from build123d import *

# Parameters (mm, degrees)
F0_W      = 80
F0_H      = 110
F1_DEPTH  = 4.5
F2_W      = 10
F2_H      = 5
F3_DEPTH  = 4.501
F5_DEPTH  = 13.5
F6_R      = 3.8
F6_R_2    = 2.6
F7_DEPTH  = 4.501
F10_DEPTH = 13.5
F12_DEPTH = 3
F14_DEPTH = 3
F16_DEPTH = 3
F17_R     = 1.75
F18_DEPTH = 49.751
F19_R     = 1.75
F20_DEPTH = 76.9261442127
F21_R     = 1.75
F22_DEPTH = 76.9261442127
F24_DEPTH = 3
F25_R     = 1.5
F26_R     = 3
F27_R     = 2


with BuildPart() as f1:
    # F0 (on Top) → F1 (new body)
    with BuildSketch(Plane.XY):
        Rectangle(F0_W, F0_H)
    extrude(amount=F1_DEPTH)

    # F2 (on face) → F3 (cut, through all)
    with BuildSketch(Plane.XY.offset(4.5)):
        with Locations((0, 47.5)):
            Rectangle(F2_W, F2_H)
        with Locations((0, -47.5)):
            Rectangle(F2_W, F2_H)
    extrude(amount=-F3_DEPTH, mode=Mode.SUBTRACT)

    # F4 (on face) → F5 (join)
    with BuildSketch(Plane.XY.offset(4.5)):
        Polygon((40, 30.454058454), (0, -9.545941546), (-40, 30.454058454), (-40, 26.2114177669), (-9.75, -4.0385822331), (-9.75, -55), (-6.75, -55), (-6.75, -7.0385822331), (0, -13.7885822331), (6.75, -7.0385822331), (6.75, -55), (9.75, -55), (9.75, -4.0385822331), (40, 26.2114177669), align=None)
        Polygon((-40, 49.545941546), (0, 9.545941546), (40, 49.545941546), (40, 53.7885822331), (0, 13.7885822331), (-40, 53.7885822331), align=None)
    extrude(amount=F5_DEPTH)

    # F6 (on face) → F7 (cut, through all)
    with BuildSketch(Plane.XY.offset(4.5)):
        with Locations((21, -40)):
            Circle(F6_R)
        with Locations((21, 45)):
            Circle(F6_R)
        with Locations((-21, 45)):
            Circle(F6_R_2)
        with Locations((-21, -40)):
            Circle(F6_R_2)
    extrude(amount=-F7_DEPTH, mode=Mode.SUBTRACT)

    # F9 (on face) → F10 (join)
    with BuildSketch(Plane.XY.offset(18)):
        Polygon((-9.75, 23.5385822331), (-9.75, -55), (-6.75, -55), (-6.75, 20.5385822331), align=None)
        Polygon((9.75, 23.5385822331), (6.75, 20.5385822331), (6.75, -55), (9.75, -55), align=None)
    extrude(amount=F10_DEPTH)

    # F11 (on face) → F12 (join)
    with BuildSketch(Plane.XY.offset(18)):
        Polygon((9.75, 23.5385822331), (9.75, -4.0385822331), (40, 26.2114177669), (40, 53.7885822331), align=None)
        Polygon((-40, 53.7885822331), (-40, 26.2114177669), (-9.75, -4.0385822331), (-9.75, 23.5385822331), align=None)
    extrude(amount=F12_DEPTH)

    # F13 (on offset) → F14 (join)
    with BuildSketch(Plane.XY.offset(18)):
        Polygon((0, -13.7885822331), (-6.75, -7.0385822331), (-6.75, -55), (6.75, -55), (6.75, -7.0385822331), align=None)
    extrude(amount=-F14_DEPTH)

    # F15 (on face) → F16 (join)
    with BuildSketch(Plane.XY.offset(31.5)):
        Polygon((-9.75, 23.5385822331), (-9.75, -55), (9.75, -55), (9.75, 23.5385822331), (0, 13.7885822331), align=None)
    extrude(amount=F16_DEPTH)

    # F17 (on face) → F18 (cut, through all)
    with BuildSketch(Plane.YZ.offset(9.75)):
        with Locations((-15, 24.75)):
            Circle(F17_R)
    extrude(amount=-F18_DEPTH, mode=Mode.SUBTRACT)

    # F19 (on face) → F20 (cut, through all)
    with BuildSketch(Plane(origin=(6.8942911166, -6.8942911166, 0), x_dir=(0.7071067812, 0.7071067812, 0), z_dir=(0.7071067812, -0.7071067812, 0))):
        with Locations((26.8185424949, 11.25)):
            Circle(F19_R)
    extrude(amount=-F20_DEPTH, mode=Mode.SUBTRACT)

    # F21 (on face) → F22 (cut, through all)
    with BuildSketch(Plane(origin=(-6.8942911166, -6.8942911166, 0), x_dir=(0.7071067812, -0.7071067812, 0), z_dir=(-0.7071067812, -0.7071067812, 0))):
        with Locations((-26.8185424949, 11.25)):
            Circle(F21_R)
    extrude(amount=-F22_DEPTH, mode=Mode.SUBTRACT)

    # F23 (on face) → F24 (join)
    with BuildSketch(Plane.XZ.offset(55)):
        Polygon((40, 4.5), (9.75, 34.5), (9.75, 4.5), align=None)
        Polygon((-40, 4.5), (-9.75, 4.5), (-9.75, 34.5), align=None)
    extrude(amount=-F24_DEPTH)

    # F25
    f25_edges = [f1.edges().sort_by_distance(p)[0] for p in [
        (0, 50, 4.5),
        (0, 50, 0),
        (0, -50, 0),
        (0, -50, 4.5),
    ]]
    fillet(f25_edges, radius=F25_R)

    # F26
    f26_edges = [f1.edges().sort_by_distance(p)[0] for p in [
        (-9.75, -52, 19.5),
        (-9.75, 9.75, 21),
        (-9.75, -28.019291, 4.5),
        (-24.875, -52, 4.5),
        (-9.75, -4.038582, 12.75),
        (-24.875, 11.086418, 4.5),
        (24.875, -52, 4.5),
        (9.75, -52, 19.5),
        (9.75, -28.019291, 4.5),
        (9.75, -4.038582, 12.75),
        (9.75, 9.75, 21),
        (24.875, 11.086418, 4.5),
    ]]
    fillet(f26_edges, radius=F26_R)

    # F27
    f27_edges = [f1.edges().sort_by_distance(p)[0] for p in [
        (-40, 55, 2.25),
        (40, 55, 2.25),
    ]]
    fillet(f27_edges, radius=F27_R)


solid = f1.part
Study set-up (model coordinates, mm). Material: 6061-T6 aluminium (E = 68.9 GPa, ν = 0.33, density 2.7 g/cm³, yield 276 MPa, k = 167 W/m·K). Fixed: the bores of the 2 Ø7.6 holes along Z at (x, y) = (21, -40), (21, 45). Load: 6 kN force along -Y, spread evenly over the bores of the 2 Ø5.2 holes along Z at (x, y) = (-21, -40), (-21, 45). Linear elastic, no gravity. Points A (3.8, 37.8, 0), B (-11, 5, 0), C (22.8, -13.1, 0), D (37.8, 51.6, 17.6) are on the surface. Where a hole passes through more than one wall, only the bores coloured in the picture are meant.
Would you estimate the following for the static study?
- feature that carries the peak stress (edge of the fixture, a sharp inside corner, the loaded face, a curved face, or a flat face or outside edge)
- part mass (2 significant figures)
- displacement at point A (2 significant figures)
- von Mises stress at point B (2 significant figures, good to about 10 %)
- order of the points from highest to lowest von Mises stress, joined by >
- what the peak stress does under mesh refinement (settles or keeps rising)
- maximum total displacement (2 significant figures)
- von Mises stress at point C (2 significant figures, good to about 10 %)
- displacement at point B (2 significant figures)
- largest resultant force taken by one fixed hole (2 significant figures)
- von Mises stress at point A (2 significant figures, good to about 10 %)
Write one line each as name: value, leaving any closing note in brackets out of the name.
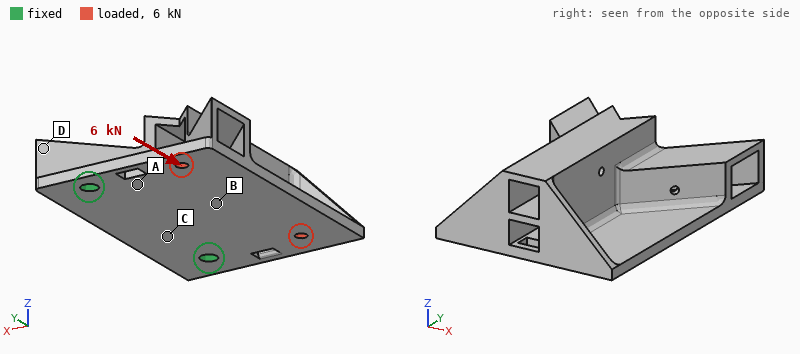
feature that carries the peak stress: edge of the fixture
part mass: 200 g
displacement at point A: 13 µm
von Mises stress at point B: 22 MPa
order of the points from highest to lowest von Mises stress, joined by >: A > B > C > D
what the peak stress does under mesh refinement: keeps rising
maximum total displacement: 54 µm
von Mises stress at point C: 12 MPa
displacement at point B: 22 µm
largest resultant force taken by one fixed hole: 4.2 kN
von Mises stress at point A: 33 MPa
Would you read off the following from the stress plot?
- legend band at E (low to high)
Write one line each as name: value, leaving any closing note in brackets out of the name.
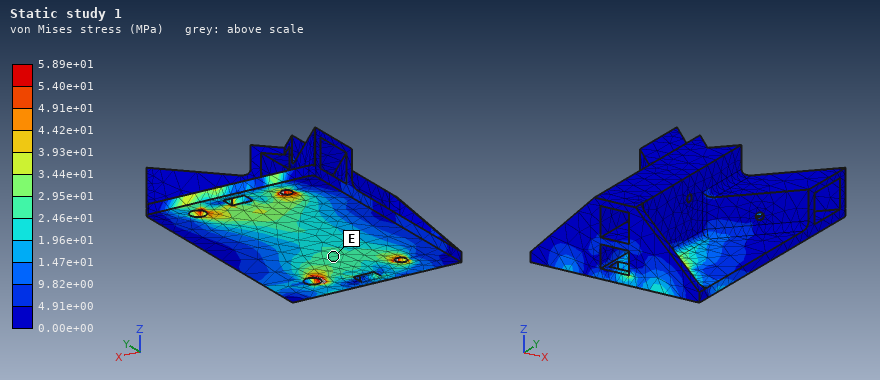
legend band at E: 2.46e+01 to 2.95e+01 MPa
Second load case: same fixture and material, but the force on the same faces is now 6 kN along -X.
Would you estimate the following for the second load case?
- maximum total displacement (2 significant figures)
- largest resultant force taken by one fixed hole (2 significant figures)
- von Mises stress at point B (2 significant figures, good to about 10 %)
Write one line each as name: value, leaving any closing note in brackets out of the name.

maximum total displacement: 26 µm
largest resultant force taken by one fixed hole: 3.0 kN
von Mises stress at point B: 4.3 MPa
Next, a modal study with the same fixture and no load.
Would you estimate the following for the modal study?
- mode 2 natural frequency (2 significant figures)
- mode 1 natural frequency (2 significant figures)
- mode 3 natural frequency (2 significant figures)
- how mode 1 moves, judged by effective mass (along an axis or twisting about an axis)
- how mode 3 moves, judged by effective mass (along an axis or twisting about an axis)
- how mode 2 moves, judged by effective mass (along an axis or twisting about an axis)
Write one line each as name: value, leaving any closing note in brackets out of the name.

mode 2 natural frequency: 3400 Hz
mode 1 natural frequency: 1000 Hz
mode 3 natural frequency: 5000 Hz
how mode 1 moves, judged by effective mass: along Z
how mode 3 moves, judged by effective mass: along Z
how mode 2 moves, judged by effective mass: twisting about X
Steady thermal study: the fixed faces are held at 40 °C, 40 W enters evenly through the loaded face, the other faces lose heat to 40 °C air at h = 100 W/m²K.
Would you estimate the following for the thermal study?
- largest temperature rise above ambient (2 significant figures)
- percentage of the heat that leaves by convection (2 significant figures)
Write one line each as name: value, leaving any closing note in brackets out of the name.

largest temperature rise above ambient: 21 K
percentage of the heat that leaves by convection: 59 %
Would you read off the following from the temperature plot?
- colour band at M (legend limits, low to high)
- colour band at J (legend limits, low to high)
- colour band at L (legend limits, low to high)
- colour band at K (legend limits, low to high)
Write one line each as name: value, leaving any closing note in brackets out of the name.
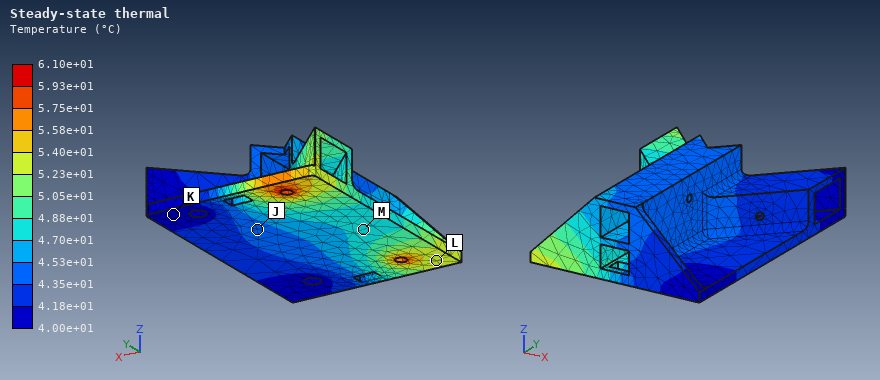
colour band at M: 4.70e+01 to 4.88e+01 °C
colour band at J: 4.35e+01 to 4.53e+01 °C
colour band at L: 5.23e+01 to 5.40e+01 °C
colour band at K: 4.00e+01 to 4.18e+01 °C
